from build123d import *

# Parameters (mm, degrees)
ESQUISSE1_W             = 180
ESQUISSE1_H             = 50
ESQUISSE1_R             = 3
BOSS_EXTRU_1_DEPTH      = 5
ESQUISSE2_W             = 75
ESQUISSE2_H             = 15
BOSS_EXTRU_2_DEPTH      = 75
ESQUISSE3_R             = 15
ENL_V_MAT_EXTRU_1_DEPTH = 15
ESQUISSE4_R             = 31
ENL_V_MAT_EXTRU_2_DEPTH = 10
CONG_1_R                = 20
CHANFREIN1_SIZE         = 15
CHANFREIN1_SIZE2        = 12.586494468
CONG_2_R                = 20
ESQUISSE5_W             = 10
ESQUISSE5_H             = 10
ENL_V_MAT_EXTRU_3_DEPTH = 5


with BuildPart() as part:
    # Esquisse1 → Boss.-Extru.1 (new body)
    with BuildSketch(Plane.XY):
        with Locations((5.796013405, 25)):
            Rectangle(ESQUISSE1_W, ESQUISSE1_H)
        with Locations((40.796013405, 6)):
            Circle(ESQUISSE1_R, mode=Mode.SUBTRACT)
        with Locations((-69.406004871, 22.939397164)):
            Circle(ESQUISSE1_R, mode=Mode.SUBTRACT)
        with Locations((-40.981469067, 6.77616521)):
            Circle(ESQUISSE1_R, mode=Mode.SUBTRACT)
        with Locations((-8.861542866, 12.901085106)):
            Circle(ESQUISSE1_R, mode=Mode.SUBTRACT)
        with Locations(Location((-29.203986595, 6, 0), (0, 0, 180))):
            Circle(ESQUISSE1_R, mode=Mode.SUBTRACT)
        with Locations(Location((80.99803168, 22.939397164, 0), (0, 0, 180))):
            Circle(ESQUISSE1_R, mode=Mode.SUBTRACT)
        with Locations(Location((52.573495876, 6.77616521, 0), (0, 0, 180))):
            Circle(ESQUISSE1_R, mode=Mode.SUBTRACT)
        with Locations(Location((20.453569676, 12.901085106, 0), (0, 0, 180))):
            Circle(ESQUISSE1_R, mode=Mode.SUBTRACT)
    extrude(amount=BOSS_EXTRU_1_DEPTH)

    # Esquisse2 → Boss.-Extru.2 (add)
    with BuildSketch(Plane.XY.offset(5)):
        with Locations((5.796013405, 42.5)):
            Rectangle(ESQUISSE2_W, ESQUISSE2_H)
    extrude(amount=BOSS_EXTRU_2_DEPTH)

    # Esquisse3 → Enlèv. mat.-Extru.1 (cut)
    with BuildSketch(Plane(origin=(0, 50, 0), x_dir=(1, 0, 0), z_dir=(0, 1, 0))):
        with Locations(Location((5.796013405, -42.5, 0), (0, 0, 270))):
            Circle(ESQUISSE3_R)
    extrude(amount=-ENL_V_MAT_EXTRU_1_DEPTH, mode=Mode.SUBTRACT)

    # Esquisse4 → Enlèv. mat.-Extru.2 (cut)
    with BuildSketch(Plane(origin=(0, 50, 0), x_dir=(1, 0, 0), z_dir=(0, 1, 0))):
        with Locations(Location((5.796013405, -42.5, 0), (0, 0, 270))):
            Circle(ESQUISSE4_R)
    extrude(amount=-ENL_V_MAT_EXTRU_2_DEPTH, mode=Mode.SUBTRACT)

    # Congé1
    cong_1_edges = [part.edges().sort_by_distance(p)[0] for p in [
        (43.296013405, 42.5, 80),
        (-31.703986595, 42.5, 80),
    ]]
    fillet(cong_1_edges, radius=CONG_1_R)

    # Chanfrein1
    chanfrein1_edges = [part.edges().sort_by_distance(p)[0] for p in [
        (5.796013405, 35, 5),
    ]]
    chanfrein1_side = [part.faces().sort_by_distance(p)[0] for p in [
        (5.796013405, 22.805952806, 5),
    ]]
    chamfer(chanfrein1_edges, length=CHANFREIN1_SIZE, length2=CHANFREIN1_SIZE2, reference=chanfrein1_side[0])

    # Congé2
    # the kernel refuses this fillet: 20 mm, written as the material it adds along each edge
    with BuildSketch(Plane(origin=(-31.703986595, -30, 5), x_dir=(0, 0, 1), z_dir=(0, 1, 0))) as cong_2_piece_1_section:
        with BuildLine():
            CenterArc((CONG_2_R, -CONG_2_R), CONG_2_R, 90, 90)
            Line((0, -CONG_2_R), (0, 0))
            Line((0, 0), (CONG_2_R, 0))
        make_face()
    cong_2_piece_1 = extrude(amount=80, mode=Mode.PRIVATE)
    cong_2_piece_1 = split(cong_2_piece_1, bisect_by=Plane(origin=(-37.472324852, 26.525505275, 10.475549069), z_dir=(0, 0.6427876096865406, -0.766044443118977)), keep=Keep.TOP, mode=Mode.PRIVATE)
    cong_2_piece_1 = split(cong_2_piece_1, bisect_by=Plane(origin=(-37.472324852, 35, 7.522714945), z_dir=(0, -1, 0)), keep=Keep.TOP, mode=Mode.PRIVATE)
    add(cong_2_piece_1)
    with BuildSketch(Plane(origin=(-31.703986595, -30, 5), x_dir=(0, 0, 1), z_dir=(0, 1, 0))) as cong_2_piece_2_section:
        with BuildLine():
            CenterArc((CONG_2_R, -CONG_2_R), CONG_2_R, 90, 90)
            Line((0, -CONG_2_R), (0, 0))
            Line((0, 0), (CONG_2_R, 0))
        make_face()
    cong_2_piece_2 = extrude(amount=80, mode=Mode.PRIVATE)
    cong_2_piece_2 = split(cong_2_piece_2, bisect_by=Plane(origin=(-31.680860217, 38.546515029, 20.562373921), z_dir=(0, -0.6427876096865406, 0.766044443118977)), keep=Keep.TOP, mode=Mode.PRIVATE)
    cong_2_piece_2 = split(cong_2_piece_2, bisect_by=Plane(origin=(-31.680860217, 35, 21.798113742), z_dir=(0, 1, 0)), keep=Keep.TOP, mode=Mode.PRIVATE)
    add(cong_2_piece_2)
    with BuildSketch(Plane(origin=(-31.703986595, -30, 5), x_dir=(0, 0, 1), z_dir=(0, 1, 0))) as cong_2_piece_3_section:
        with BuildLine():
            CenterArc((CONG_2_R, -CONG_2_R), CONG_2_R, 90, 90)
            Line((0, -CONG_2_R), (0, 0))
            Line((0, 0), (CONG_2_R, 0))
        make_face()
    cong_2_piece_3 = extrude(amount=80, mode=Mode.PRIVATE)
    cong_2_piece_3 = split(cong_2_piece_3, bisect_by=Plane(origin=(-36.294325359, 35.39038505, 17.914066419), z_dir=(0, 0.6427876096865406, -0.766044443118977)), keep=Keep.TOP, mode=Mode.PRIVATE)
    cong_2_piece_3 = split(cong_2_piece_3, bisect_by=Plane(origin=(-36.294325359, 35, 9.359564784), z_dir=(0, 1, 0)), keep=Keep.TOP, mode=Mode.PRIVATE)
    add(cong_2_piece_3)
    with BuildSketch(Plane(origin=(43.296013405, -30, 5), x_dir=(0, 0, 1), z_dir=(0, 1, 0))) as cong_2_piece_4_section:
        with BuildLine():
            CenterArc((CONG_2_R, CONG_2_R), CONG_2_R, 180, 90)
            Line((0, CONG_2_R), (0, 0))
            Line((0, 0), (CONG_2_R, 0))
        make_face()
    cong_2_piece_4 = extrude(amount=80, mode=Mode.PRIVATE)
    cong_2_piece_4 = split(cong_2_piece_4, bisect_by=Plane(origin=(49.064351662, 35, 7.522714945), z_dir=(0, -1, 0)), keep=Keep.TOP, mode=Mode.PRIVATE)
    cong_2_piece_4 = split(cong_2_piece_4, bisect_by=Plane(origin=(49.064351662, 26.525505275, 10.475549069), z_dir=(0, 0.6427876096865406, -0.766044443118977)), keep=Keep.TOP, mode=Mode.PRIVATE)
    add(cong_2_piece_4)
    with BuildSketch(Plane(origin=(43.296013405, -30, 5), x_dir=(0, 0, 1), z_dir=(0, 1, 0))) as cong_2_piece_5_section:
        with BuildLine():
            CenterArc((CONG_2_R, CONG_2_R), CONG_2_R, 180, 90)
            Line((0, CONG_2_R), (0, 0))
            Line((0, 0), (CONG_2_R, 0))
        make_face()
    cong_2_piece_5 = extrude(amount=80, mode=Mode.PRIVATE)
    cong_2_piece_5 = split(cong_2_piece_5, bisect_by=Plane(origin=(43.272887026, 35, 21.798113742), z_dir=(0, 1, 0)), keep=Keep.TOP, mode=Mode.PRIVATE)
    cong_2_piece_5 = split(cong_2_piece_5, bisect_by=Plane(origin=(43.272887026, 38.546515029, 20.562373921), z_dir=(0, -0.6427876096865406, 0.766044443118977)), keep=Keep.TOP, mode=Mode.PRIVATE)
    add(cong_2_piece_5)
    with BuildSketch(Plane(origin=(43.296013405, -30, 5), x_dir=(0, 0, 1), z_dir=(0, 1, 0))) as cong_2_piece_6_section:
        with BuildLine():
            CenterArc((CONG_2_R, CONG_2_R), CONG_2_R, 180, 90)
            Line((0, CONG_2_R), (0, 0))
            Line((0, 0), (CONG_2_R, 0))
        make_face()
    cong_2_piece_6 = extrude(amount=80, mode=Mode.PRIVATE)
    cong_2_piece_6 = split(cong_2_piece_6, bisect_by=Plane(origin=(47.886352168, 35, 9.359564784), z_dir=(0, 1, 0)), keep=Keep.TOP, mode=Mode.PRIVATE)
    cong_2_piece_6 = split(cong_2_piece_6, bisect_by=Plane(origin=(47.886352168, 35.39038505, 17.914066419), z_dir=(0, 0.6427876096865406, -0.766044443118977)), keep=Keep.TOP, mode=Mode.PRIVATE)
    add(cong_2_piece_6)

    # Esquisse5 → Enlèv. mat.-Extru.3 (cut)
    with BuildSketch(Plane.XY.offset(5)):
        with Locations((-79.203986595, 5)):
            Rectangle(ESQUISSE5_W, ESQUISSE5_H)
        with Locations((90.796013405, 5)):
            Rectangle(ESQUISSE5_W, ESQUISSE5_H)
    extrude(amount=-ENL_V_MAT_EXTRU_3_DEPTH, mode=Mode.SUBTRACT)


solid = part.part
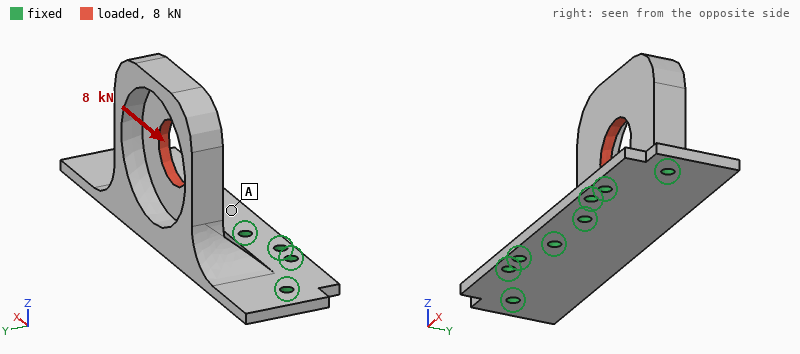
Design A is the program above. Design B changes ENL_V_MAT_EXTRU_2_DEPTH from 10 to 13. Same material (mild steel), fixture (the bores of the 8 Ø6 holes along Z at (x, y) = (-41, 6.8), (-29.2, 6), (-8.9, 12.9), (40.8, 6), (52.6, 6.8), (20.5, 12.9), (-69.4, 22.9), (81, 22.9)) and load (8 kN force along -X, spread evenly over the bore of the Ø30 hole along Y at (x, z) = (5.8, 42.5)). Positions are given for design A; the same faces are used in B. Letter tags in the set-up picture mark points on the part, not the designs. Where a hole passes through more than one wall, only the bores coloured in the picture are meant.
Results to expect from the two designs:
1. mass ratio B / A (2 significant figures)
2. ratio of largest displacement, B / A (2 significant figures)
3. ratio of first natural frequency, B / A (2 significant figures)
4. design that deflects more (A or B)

0.93
1.2
1.1
B
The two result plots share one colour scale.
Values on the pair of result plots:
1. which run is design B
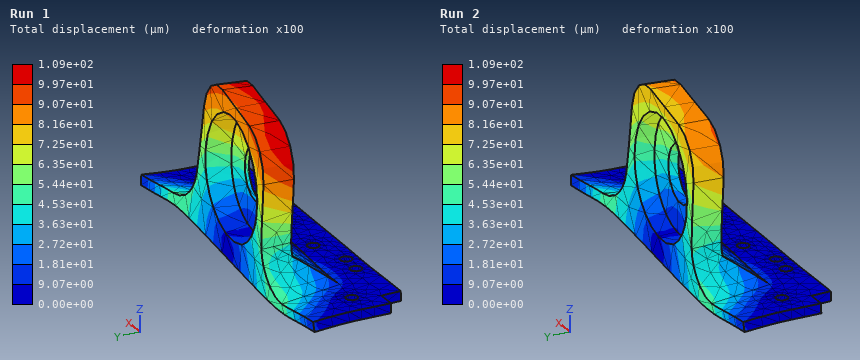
Run 1
